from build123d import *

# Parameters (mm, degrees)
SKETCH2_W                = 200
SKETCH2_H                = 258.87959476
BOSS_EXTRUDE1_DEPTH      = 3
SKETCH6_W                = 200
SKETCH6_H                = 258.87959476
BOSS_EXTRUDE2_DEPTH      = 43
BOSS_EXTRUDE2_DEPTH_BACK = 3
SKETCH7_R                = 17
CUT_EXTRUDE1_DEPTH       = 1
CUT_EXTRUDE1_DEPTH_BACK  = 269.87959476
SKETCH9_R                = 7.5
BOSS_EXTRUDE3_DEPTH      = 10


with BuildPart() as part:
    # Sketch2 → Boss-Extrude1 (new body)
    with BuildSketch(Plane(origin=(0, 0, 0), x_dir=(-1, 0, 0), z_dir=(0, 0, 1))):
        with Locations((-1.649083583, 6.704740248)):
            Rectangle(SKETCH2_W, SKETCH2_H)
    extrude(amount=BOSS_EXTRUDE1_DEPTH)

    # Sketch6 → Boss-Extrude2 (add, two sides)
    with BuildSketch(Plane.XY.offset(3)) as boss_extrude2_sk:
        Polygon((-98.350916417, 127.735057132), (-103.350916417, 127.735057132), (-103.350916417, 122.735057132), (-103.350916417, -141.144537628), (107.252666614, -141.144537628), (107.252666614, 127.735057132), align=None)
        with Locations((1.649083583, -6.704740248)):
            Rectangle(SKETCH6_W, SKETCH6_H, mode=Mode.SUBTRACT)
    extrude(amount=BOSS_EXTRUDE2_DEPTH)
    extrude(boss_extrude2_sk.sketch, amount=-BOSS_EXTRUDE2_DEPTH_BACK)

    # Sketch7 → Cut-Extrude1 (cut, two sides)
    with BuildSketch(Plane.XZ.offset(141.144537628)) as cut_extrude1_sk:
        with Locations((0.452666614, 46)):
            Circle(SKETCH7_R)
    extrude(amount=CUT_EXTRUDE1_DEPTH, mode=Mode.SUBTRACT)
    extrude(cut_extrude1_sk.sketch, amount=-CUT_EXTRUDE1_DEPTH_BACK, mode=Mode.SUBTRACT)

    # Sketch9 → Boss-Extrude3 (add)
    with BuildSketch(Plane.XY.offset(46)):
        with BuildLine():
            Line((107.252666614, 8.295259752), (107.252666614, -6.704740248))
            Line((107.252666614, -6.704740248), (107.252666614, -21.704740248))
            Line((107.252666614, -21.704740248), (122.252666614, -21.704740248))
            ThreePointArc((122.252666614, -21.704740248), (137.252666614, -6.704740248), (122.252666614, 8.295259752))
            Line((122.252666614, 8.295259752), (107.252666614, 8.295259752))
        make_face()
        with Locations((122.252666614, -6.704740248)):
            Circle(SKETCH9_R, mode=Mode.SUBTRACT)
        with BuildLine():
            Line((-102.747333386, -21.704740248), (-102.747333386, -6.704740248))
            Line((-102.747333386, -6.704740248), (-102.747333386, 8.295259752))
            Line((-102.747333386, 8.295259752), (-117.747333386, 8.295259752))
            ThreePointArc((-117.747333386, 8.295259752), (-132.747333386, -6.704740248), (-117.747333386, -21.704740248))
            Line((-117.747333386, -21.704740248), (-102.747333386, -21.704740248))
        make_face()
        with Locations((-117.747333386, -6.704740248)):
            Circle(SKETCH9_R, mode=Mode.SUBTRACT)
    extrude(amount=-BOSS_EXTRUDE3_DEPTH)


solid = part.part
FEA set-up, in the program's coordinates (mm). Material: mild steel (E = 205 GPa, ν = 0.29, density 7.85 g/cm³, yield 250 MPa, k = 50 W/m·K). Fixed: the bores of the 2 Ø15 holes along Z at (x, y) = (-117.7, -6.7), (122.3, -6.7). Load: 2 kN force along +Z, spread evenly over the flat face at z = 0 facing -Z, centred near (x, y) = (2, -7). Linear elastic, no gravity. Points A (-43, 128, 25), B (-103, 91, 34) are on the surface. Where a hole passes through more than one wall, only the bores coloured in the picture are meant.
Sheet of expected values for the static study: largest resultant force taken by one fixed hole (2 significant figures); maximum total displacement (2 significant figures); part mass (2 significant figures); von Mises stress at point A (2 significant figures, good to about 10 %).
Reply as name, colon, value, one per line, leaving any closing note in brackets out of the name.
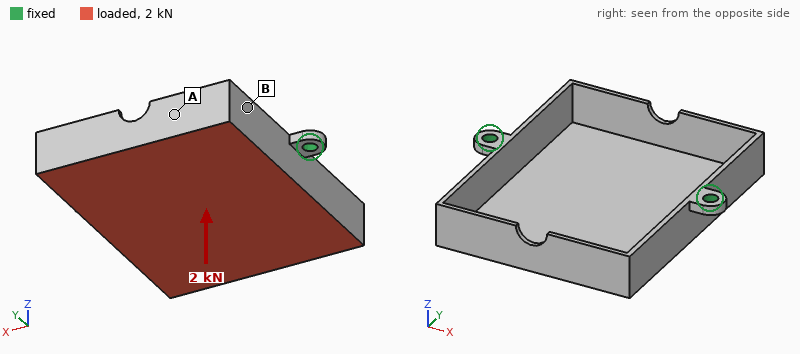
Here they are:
largest resultant force taken by one fixed hole: 1.1 kN
maximum total displacement: 0.26 mm
part mass: 3.0 kg
von Mises stress at point A: 8.7 MPa
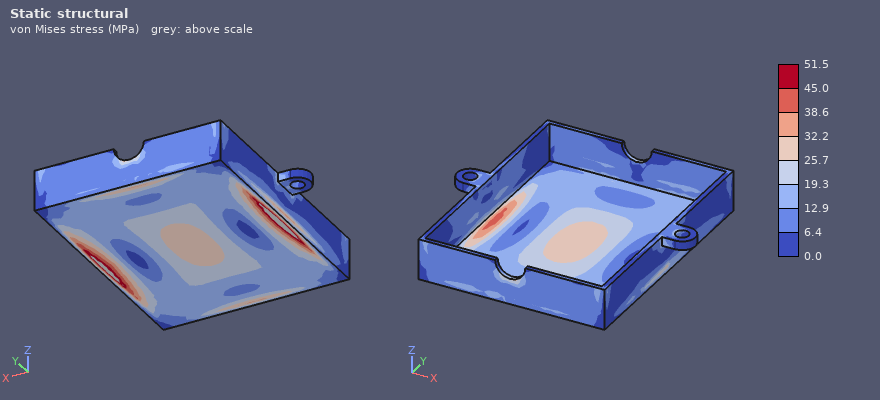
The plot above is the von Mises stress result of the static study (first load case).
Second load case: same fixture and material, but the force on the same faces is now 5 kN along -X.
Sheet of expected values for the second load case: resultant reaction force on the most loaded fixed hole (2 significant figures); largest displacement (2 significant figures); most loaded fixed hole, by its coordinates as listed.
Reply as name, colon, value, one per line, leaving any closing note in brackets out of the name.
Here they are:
resultant reaction force on the most loaded fixed hole: 2.8 kN
largest displacement: 0.23 mm
most loaded fixed hole, by its coordinates as listed: (122.3, -6.7)
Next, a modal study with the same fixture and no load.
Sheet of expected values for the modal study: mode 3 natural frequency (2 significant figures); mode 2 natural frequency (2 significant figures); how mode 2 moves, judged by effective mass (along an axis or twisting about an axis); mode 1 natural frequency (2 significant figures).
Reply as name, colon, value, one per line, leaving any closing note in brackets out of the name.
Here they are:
mode 3 natural frequency: 480 Hz
mode 2 natural frequency: 420 Hz
how mode 2 moves, judged by effective mass: twisting about Z
mode 1 natural frequency: 320 Hz
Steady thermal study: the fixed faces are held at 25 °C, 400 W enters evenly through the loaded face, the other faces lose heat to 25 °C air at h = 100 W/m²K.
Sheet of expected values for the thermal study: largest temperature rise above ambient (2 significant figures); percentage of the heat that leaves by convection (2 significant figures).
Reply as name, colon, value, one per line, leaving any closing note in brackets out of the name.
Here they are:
largest temperature rise above ambient: 63 K
percentage of the heat that leaves by convection: 97 %
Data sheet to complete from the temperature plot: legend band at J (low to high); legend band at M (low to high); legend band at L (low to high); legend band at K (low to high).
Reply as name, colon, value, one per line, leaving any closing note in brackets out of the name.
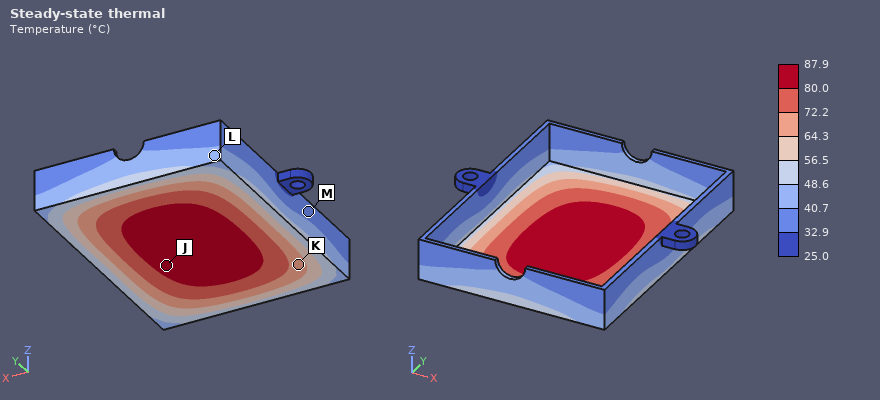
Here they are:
legend band at J: 80.0 to 87.9 °C
legend band at M: 32.9 to 40.7 °C
legend band at L: 40.7 to 48.6 °C
legend band at K: 64.3 to 72.2 °C
